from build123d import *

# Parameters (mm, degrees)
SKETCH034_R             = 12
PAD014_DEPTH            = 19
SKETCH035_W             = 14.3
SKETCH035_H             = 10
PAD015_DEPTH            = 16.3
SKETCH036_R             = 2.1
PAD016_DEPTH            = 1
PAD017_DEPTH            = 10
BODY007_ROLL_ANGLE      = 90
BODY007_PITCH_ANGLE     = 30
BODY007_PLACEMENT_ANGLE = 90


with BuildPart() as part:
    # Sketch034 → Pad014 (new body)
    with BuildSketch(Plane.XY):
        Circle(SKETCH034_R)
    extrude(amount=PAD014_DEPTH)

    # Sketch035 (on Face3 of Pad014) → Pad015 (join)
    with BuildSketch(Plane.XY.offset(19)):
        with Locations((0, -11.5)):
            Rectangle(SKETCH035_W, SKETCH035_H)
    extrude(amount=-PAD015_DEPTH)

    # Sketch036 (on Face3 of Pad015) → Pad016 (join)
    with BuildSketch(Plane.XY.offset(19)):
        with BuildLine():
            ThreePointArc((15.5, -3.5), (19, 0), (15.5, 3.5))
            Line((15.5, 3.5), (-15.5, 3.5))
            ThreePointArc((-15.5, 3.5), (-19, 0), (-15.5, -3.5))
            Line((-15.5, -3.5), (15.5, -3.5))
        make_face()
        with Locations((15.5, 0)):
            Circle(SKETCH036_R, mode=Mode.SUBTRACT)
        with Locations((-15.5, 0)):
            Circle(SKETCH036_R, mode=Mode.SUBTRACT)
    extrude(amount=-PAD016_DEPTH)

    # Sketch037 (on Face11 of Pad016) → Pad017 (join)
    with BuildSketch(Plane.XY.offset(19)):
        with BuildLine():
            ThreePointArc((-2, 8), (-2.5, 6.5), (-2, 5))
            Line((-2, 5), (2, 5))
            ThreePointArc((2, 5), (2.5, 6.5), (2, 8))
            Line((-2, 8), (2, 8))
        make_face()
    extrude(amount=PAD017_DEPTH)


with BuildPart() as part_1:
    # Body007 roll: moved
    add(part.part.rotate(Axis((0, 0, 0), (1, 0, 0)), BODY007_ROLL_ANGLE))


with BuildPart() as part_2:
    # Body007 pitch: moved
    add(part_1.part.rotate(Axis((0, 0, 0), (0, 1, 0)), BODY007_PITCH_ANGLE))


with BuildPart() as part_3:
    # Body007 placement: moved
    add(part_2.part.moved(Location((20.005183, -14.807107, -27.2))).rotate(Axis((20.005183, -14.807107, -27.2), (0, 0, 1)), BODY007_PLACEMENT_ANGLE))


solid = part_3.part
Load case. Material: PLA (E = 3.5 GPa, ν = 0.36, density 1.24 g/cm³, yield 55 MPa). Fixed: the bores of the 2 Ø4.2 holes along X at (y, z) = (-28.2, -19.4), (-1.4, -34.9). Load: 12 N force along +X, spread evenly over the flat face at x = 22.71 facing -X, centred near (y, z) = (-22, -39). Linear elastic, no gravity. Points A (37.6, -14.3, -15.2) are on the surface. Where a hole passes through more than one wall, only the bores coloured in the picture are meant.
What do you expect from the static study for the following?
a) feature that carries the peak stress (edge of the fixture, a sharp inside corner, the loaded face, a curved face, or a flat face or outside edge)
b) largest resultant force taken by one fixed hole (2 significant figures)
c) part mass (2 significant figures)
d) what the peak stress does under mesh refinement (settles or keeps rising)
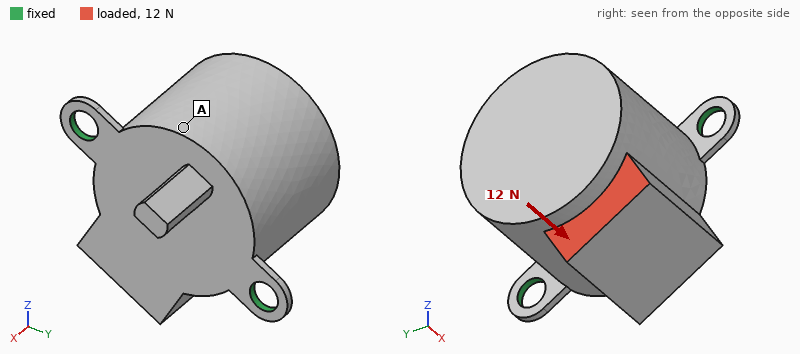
edge of the fixture
7.2 N
12 g
keeps rising
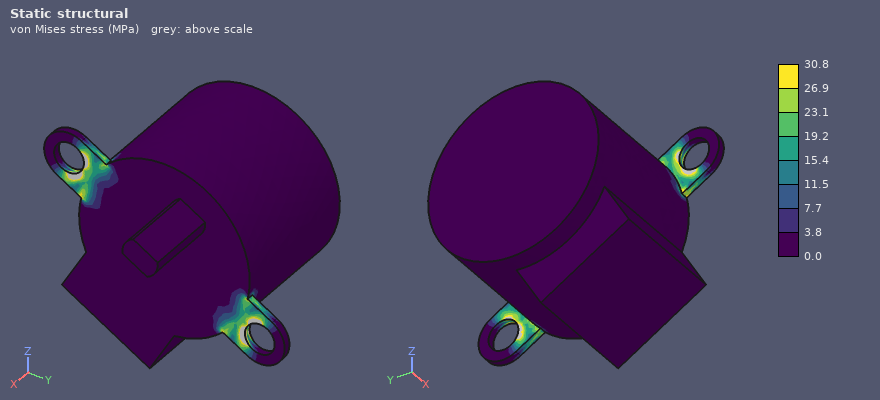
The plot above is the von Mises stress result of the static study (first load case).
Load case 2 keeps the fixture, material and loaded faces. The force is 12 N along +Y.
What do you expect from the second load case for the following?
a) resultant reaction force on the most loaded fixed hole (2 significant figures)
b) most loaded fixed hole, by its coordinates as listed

12 N
(-1.4, -34.9)
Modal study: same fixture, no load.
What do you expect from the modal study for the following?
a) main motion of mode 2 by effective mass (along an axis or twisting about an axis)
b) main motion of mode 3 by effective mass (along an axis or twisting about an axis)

along X
along Y
